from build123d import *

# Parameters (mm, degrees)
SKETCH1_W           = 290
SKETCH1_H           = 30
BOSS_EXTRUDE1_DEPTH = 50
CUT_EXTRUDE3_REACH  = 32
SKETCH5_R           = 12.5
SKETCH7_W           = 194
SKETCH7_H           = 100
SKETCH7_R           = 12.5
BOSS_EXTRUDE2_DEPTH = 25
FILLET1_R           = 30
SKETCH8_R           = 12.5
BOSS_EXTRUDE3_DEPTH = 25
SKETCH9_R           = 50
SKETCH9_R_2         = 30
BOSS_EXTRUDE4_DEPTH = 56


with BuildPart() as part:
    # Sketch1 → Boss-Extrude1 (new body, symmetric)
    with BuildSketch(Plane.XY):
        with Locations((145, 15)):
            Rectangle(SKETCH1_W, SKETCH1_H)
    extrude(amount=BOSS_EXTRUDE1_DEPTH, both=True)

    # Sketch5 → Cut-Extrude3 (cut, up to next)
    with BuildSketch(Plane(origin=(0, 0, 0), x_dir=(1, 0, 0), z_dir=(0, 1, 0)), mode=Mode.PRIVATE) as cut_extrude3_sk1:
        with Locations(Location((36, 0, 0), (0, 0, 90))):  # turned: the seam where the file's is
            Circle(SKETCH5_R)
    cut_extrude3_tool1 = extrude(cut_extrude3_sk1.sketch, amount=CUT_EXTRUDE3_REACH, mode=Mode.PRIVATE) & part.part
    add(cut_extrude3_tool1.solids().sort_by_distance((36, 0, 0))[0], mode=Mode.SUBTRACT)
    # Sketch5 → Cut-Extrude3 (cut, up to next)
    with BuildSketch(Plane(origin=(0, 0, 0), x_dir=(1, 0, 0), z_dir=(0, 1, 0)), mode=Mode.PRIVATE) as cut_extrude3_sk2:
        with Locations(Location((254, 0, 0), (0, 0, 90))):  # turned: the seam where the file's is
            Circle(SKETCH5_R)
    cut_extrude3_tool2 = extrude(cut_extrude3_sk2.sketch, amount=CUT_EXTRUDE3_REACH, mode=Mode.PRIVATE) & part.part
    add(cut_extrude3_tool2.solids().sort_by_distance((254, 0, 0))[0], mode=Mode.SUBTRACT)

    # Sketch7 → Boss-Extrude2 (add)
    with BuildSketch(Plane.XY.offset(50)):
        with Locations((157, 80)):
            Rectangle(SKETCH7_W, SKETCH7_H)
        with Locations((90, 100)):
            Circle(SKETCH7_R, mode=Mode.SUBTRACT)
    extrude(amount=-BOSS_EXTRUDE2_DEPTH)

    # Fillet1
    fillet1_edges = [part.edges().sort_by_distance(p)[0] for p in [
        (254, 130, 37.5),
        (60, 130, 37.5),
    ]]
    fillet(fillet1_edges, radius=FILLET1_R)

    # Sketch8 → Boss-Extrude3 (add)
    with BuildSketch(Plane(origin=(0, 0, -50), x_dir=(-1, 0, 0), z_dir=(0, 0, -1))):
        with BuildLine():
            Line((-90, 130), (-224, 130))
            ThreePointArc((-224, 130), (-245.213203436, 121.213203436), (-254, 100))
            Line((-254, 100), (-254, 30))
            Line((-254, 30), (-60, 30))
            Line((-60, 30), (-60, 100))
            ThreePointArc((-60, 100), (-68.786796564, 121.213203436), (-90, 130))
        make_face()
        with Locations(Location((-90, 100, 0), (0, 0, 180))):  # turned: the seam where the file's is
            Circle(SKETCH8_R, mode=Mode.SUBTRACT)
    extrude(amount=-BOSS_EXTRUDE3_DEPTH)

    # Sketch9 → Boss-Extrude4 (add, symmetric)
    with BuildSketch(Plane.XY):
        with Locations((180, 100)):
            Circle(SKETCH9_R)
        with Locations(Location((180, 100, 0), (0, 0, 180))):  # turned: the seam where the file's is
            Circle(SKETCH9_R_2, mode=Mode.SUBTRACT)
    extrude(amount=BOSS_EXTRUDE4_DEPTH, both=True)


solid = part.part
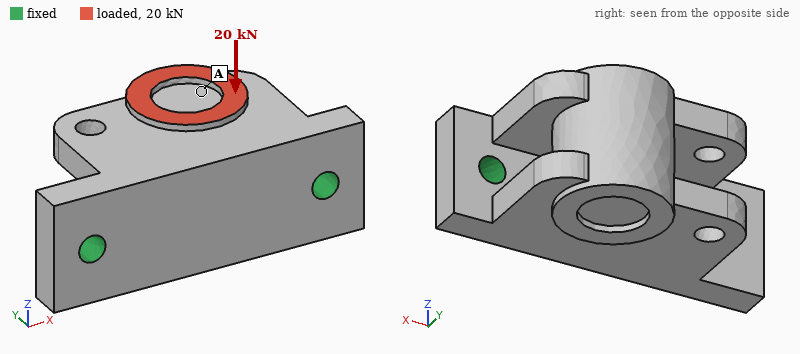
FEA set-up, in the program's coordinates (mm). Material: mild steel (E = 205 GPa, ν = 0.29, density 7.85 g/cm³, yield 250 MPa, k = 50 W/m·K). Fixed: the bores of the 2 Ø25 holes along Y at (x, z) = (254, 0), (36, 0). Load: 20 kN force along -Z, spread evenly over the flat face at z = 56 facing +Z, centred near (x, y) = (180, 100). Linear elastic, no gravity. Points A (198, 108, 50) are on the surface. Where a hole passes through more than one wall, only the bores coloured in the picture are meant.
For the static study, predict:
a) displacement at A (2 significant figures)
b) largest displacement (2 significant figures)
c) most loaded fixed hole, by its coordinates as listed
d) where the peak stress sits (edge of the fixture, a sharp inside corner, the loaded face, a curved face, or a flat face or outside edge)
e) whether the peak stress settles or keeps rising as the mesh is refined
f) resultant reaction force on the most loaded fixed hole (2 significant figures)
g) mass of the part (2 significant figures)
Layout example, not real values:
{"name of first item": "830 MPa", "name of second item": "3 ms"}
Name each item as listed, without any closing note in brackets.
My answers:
{"displacement at A": "53 µm", "largest displacement": "71 µm", "most loaded fixed hole, by its coordinates as listed": "(254, 0)", "where the peak stress sits": "edge of the fixture", "whether the peak stress settles or keeps rising as the mesh is refined": "keeps rising", "resultant reaction force on the most loaded fixed hole": "14 kN", "mass of the part": "17 kg"}
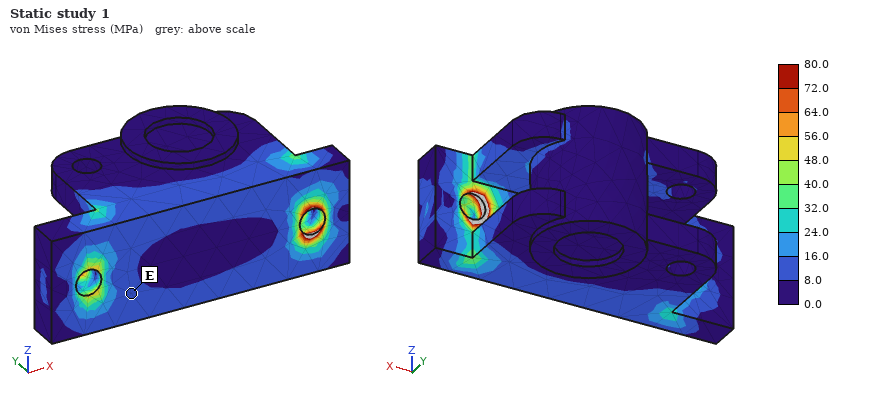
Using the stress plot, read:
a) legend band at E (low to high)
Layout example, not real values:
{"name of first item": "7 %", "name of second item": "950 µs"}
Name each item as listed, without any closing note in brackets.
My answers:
{"legend band at E": "8.0 to 16.0 MPa"}
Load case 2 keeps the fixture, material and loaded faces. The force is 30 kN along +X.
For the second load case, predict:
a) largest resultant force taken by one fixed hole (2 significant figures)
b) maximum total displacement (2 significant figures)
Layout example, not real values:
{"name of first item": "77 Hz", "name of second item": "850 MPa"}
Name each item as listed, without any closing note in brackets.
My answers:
{"largest resultant force taken by one fixed hole": "21 kN", "maximum total displacement": "21 µm"}
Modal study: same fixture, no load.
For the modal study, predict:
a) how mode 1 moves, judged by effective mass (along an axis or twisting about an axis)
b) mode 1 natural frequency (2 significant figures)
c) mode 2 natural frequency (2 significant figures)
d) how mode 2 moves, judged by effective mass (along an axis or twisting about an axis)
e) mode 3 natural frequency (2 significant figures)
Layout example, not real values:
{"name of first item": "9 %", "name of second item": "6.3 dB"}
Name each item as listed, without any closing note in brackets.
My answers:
{"how mode 1 moves, judged by effective mass": "along Z", "mode 1 natural frequency": "1100 Hz", "mode 2 natural frequency": "2700 Hz", "how mode 2 moves, judged by effective mass": "along Y", "mode 3 natural frequency": "3200 Hz"}
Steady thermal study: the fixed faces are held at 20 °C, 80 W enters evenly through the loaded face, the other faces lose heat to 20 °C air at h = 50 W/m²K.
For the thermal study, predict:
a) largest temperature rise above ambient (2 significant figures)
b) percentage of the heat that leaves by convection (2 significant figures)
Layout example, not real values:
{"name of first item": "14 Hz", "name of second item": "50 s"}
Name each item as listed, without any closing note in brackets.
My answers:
{"largest temperature rise above ambient": "20 K", "percentage of the heat that leaves by convection": "67 %"}
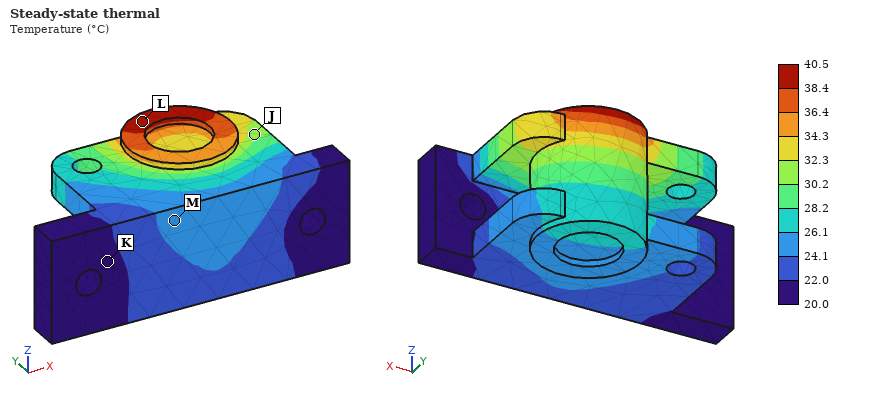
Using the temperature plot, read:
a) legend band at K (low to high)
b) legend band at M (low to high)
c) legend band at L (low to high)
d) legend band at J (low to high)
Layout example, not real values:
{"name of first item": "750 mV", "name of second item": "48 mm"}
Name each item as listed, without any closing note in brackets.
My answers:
{"legend band at K": "20.0 to 22.0 °C", "legend band at M": "24.1 to 26.1 °C", "legend band at L": "38.4 to 40.5 °C", "legend band at J": "30.2 to 32.3 °C"}
